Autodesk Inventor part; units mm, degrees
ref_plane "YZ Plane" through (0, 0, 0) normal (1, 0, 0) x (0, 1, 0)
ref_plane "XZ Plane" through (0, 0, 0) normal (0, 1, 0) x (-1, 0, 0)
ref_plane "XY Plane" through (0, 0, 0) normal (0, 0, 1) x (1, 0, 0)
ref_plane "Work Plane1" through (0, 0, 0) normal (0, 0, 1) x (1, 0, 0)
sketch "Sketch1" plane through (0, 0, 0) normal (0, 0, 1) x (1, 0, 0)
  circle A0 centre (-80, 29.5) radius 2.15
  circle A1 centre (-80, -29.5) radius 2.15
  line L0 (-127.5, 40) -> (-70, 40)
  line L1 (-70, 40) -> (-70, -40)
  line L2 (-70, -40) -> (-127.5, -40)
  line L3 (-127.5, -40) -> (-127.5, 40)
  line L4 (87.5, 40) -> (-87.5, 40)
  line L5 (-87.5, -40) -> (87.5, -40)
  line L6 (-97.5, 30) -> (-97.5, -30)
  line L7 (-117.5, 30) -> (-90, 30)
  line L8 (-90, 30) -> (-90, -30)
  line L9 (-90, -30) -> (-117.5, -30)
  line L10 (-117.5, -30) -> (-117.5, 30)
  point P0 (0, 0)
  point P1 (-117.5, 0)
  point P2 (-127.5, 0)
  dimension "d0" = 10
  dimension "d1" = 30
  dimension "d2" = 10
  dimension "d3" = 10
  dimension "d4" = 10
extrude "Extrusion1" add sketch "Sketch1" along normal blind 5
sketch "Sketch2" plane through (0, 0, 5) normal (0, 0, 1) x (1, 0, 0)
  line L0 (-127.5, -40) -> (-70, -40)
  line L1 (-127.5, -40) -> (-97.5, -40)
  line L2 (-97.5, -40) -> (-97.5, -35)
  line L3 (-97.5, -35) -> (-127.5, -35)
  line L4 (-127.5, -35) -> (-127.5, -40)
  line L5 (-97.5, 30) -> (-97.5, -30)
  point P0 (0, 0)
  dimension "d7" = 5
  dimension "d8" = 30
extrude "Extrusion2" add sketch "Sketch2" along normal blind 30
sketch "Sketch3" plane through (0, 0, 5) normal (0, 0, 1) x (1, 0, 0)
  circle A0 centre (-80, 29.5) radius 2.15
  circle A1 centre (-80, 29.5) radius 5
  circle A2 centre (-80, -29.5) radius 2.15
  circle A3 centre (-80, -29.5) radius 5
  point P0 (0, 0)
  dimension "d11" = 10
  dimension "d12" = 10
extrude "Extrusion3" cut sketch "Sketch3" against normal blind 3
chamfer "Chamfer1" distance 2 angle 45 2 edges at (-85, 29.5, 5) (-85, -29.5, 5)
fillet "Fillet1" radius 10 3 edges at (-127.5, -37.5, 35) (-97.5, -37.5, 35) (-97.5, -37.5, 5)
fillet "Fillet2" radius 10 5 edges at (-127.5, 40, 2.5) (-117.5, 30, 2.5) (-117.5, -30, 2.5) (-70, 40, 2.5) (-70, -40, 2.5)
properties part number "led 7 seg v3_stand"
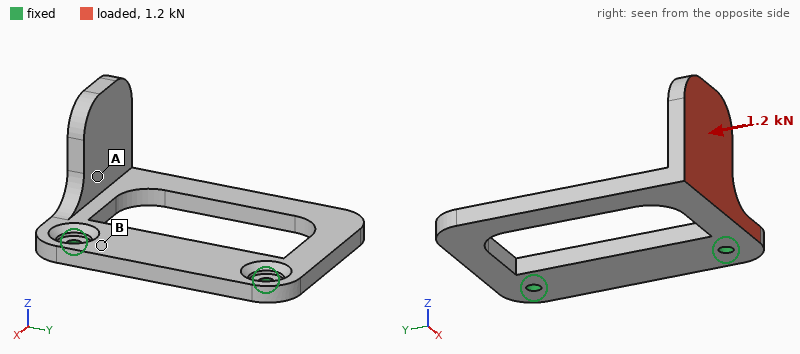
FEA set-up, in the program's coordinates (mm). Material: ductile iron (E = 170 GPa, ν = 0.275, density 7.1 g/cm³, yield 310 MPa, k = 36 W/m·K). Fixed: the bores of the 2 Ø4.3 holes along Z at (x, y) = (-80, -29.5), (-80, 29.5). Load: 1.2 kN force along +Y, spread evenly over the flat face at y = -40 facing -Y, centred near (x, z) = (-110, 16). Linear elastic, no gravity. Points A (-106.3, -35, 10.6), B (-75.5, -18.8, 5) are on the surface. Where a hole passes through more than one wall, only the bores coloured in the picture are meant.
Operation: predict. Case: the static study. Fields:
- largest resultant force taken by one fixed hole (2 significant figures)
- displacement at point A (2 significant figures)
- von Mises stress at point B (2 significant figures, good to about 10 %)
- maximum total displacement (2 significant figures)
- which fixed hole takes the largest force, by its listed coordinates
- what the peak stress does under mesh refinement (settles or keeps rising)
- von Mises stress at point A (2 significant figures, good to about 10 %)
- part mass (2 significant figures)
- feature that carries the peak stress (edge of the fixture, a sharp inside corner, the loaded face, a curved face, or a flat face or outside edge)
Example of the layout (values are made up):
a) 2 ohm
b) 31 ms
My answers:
a) 1.3 kN
b) 0.15 mm
c) 34 MPa
d) 0.49 mm
e) (-80, 29.5)
f) keeps rising
g) 75 MPa
h) 130 g
i) edge of the fixture
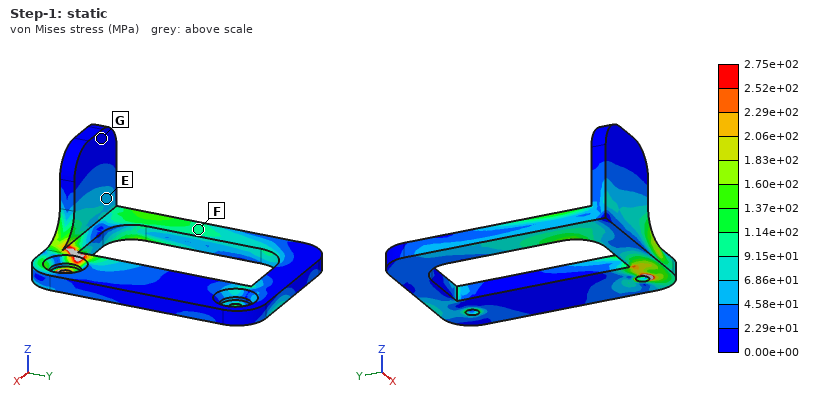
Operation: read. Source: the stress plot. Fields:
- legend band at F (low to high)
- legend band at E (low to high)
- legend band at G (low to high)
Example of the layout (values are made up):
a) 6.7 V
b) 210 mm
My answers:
a) 9.15e+01 to 1.14e+02 MPa
b) 4.58e+01 to 6.86e+01 MPa
c) 0.00e+00 to 2.29e+01 MPa
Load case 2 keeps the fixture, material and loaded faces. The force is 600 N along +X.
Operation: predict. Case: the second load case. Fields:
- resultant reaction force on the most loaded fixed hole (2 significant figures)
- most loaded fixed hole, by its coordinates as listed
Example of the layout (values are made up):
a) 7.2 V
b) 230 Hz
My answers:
a) 670 N
b) (-80, -29.5)
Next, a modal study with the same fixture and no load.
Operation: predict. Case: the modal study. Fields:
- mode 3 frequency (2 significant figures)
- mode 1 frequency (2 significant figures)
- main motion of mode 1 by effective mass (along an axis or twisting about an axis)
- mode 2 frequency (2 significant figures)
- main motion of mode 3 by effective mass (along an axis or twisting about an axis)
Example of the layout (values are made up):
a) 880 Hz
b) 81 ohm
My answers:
a) 2000 Hz
b) 630 Hz
c) along Z
d) 1300 Hz
e) along Y
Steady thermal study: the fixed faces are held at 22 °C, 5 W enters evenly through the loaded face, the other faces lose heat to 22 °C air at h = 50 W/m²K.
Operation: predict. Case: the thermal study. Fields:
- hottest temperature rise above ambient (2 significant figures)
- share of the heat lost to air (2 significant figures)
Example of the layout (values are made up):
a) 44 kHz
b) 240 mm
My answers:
a) 26 K
b) 67 %
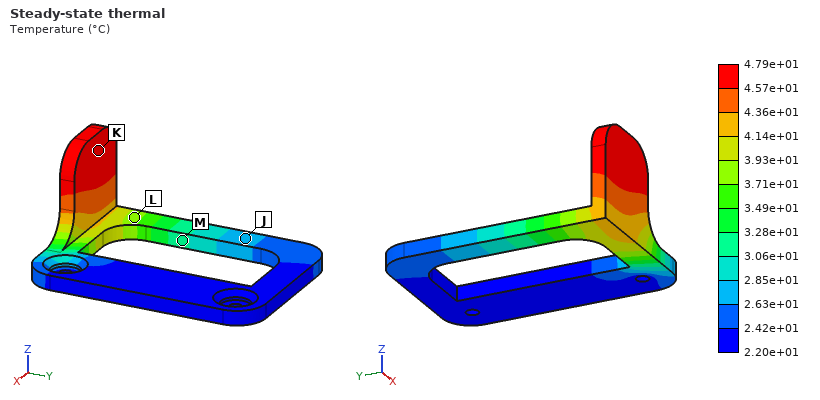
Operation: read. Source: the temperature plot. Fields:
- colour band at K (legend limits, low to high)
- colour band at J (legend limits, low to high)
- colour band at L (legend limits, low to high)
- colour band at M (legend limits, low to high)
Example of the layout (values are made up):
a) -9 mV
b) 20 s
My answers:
a) 4.57e+01 to 4.79e+01 °C
b) 2.63e+01 to 2.85e+01 °C
c) 3.71e+01 to 3.93e+01 °C
d) 3.06e+01 to 3.28e+01 °C
